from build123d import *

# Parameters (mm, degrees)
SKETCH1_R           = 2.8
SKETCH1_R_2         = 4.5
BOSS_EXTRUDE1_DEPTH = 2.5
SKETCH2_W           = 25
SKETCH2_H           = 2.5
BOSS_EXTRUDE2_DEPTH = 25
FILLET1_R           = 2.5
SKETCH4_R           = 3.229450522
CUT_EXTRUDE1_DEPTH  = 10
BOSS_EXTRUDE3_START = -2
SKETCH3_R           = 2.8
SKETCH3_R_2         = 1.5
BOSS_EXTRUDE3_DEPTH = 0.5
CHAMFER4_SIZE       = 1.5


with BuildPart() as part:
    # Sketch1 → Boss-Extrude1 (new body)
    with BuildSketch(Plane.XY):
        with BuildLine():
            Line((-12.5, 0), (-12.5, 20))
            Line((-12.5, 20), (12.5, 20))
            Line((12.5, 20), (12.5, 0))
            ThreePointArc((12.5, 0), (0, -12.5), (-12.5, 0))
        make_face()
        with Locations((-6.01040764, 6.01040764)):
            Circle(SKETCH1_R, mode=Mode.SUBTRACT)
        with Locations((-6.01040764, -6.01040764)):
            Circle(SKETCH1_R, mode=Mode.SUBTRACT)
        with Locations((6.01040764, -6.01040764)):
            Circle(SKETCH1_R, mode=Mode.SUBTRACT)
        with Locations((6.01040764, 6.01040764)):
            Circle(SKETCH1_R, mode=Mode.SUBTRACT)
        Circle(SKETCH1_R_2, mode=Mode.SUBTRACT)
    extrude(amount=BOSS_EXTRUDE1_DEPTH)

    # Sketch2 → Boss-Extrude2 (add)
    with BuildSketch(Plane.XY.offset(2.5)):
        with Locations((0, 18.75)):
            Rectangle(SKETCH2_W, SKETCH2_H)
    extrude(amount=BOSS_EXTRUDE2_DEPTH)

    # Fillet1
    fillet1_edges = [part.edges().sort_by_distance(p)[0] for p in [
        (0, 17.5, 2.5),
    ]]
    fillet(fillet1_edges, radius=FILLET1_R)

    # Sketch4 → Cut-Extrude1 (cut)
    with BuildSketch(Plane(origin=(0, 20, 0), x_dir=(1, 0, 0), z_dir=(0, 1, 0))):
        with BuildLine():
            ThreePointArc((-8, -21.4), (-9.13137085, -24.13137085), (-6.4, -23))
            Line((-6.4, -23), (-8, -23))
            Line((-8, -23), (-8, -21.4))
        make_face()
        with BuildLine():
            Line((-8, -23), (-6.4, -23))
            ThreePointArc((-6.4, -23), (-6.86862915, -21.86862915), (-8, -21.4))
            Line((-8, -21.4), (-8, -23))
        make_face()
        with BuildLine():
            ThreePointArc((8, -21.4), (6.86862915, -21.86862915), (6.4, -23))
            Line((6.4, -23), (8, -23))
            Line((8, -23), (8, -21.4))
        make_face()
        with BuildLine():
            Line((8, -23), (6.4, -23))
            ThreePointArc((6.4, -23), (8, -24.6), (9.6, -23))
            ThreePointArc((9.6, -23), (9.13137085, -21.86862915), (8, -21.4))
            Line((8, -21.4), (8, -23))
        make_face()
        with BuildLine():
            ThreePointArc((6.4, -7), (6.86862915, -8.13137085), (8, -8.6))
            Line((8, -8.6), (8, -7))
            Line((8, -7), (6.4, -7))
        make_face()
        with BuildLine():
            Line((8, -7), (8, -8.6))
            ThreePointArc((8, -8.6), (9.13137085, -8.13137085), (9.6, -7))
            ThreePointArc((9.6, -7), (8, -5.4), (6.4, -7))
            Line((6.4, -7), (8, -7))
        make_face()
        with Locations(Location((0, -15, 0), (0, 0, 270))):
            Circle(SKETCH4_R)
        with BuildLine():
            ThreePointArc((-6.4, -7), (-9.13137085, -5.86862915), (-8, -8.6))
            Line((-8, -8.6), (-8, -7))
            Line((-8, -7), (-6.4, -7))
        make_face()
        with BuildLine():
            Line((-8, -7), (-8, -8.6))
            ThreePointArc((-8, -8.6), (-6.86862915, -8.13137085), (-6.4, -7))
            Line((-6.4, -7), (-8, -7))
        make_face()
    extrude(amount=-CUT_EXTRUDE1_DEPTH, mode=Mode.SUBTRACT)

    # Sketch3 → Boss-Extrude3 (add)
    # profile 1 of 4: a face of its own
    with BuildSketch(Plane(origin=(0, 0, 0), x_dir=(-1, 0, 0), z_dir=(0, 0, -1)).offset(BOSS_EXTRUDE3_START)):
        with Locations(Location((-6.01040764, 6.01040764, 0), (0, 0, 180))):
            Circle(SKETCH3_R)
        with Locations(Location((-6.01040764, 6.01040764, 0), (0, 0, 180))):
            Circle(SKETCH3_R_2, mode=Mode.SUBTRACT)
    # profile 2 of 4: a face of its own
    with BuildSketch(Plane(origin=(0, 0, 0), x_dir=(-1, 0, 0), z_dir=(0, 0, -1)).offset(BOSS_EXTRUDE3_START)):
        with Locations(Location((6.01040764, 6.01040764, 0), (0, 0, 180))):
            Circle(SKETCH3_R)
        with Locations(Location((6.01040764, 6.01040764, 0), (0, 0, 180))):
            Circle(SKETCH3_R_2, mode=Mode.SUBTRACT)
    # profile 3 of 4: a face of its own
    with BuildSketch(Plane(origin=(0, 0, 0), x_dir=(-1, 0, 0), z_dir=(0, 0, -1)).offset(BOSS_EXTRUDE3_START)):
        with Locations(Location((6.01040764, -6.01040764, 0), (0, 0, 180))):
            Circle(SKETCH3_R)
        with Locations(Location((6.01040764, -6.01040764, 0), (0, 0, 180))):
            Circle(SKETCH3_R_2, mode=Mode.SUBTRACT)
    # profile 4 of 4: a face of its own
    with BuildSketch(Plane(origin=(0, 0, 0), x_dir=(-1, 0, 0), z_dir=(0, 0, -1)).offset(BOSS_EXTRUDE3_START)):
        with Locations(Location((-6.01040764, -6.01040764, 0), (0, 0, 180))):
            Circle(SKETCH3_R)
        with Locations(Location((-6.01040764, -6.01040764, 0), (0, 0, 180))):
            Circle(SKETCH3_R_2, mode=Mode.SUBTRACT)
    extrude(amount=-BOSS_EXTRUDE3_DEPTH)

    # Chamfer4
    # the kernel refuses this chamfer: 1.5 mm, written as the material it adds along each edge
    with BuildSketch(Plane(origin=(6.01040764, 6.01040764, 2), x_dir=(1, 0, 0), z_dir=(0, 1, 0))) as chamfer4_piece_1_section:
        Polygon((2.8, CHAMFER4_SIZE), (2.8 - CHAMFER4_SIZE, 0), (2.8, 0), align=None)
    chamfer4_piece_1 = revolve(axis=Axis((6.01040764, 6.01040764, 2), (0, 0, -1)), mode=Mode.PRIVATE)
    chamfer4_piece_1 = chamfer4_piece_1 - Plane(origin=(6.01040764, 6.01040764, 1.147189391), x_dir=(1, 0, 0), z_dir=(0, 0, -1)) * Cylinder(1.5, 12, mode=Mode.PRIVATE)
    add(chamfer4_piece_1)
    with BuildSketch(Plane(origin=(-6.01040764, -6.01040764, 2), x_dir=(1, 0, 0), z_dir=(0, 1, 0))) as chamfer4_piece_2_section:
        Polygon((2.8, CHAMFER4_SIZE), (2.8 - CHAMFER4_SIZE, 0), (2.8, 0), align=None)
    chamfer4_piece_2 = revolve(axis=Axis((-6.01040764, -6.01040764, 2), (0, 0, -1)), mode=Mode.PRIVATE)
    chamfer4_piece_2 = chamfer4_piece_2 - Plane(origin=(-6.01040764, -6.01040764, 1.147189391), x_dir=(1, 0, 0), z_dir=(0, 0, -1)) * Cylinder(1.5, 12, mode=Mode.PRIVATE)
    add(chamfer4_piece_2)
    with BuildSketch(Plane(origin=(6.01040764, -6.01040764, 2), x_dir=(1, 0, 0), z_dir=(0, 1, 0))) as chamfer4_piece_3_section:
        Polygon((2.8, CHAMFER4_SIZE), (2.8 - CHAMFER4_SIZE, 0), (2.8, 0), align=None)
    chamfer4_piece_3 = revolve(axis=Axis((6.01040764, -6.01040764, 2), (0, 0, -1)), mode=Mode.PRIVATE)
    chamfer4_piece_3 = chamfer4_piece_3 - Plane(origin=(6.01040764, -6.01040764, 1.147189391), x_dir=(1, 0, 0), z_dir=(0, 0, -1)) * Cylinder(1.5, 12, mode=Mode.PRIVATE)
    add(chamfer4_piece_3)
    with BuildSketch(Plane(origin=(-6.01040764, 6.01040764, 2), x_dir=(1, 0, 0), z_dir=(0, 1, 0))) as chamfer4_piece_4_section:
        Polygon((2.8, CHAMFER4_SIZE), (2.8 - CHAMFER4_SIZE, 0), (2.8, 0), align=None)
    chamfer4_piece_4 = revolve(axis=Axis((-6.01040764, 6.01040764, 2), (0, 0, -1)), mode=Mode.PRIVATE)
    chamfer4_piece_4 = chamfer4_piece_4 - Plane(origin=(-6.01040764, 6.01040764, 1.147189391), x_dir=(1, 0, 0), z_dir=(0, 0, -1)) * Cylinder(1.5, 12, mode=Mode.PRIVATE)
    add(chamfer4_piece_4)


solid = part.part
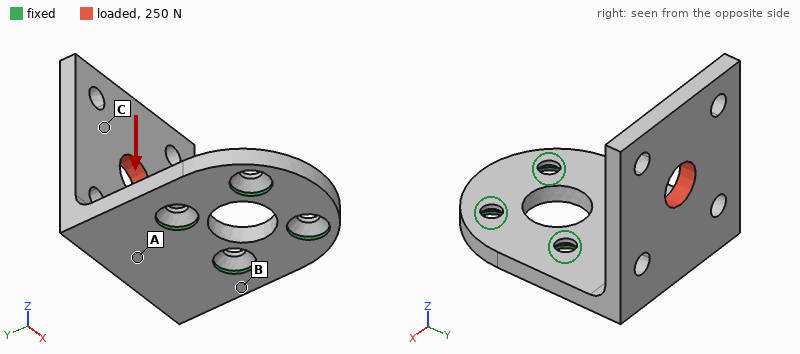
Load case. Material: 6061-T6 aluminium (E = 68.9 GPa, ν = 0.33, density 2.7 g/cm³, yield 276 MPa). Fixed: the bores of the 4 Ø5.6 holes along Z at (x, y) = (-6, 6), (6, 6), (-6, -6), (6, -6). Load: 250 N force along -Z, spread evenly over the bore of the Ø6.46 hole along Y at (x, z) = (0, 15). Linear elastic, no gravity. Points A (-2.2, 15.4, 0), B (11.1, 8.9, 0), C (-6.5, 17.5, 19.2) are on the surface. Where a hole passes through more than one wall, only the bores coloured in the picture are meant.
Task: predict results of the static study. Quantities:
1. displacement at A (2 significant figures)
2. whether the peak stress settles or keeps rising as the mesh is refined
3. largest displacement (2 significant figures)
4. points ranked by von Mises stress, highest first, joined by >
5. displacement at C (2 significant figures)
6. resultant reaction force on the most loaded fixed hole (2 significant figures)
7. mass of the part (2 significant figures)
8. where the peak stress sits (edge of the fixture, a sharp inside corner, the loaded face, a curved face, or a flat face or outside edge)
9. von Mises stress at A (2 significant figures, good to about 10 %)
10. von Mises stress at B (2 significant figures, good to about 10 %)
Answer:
0.041 mm
keeps rising
0.22 mm
B > A > C
0.15 mm
190 N
8.1 g
edge of the fixture
29 MPa
65 MPa
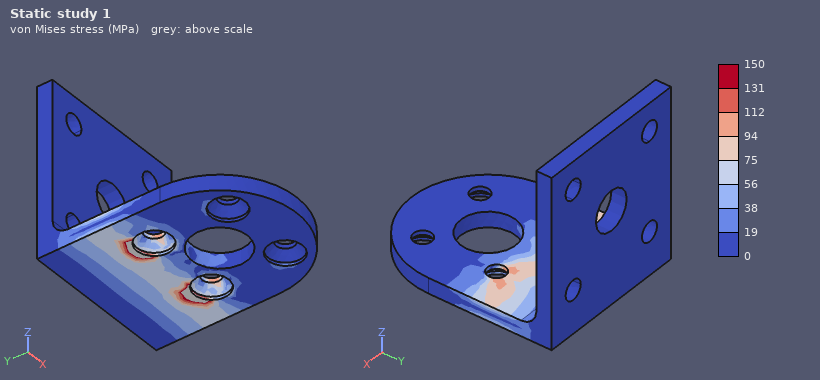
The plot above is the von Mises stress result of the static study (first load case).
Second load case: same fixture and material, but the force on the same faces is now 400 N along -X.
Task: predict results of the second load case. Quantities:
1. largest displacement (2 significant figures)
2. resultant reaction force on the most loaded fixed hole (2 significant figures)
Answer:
0.23 mm
640 N
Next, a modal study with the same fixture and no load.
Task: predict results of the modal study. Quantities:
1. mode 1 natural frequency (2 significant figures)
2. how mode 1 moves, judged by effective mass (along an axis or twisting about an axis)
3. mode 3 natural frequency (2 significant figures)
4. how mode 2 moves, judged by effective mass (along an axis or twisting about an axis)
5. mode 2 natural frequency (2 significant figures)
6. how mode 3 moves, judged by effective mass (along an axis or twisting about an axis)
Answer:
1900 Hz
along Y
6600 Hz
along X
3800 Hz
along Z
